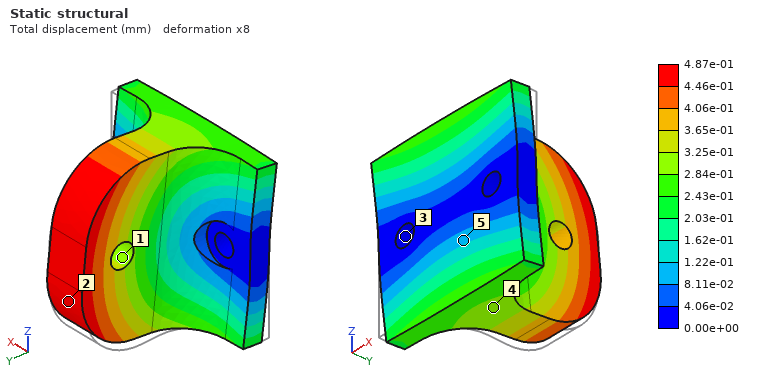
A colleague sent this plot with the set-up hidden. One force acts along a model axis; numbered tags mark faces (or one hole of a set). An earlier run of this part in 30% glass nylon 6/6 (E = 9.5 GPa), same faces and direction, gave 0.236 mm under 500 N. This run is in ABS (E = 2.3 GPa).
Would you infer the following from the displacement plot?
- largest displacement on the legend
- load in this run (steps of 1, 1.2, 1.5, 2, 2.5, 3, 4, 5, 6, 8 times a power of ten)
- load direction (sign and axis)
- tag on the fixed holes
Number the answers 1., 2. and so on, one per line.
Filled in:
1. 4.87e-01 mm
2. 250 N
3. +Z
4. 3
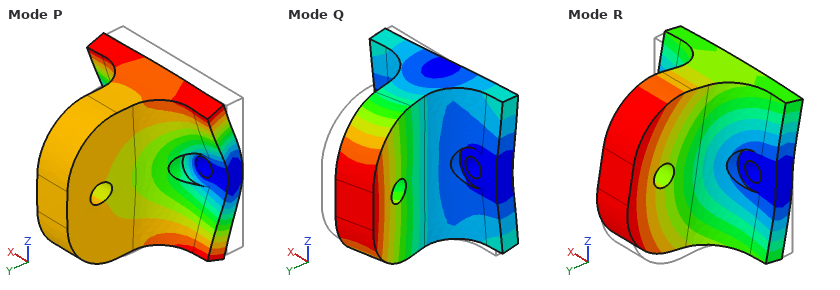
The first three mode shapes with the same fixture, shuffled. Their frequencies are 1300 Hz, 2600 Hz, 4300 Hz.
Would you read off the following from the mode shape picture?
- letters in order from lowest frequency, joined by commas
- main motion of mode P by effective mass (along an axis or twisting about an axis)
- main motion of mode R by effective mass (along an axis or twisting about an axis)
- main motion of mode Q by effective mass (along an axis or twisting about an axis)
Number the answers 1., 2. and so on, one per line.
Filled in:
1. R, Q, P
2. along Y
3. along Z
4. along X
